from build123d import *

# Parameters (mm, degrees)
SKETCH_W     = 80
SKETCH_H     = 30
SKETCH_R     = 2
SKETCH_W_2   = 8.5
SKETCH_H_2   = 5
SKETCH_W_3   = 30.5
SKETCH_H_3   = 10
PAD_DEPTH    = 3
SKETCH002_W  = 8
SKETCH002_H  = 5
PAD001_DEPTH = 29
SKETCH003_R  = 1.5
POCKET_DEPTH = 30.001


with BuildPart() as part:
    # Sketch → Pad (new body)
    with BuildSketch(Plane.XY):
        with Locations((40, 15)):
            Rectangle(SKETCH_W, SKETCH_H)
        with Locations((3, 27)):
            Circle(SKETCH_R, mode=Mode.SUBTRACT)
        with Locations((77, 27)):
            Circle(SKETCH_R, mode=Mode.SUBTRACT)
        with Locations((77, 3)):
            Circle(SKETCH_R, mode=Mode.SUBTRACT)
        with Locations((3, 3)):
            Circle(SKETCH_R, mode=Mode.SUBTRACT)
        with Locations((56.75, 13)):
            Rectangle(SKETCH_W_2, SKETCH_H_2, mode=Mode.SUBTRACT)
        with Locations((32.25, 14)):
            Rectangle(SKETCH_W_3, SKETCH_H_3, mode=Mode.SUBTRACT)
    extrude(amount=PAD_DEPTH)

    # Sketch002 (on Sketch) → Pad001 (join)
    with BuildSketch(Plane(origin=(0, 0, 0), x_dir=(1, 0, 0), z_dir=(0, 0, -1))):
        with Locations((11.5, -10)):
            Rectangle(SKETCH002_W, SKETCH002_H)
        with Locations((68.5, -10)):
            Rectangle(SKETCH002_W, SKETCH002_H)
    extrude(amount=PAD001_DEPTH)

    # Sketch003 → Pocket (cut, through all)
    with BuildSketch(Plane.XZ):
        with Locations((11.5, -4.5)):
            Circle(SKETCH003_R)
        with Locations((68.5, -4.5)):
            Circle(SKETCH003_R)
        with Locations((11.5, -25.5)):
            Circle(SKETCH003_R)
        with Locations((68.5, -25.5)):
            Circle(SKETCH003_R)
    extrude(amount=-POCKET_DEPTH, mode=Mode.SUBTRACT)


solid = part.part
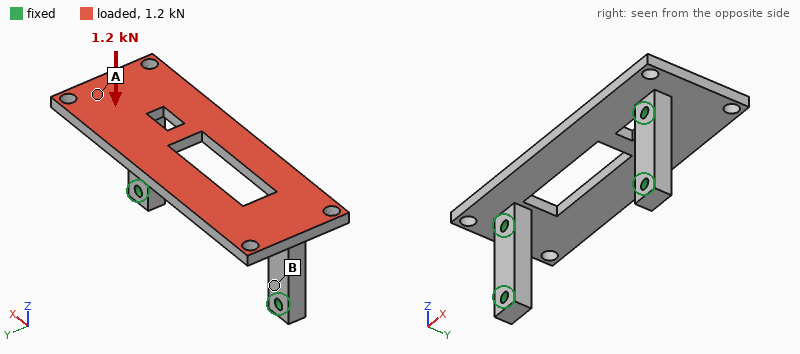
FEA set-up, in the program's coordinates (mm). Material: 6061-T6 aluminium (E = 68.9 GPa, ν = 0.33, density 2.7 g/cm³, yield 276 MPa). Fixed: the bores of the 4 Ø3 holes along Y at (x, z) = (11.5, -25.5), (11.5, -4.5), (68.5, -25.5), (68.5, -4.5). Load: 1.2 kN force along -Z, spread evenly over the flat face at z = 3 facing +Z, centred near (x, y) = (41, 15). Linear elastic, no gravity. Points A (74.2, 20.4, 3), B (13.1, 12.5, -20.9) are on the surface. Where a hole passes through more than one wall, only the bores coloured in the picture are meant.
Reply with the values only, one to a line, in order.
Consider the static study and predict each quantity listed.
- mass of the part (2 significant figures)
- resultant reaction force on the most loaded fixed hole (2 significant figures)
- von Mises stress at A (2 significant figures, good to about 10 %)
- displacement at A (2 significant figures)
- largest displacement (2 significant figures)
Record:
22 g
650 N
43 MPa
0.056 mm
0.32 mm
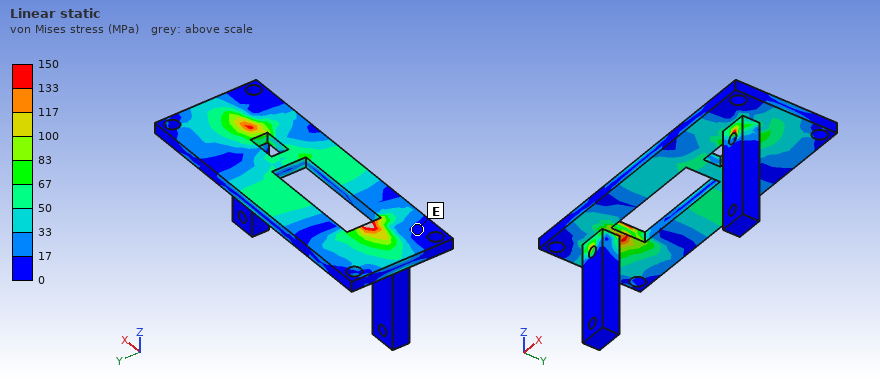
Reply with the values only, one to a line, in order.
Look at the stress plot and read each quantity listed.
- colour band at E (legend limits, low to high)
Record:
0 to 17 MPa
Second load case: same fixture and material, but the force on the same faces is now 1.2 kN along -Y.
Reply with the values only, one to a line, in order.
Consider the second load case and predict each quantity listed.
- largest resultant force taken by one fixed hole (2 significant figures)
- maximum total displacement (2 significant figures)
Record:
640 N
92 µm
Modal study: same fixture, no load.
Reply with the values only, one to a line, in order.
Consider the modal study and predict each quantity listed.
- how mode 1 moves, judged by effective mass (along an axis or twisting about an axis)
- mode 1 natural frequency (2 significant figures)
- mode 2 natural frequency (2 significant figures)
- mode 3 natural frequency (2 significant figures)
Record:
along Z
3100 Hz
5000 Hz
5500 Hz
